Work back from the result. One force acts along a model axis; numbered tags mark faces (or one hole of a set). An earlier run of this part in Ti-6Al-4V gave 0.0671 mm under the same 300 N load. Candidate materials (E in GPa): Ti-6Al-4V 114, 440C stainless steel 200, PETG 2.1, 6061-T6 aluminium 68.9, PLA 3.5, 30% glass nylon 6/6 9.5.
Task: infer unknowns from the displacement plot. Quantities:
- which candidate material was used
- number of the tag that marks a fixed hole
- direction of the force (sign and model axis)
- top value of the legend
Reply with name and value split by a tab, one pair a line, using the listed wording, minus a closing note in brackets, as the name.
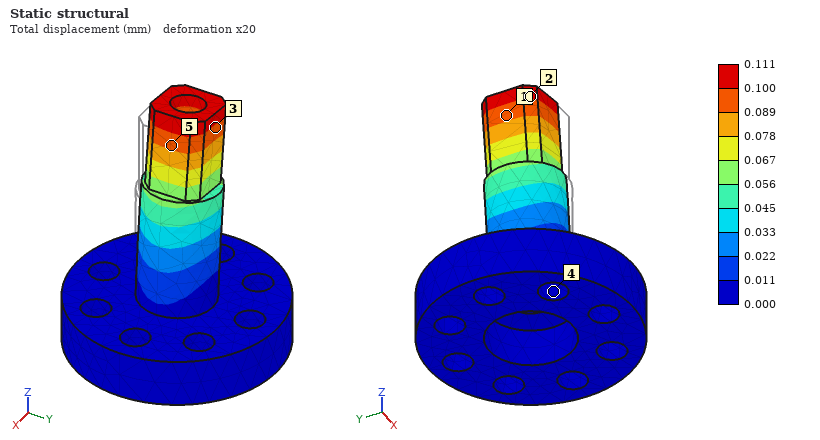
which candidate material was used	6061-T6 aluminium
number of the tag that marks a fixed hole	4
direction of the force	-X
top value of the legend	0.111 mm
